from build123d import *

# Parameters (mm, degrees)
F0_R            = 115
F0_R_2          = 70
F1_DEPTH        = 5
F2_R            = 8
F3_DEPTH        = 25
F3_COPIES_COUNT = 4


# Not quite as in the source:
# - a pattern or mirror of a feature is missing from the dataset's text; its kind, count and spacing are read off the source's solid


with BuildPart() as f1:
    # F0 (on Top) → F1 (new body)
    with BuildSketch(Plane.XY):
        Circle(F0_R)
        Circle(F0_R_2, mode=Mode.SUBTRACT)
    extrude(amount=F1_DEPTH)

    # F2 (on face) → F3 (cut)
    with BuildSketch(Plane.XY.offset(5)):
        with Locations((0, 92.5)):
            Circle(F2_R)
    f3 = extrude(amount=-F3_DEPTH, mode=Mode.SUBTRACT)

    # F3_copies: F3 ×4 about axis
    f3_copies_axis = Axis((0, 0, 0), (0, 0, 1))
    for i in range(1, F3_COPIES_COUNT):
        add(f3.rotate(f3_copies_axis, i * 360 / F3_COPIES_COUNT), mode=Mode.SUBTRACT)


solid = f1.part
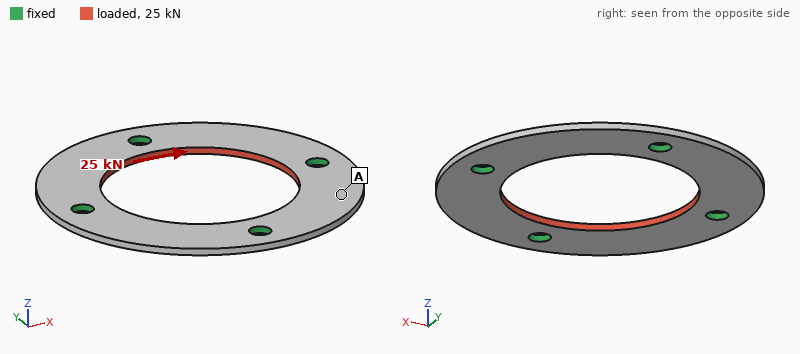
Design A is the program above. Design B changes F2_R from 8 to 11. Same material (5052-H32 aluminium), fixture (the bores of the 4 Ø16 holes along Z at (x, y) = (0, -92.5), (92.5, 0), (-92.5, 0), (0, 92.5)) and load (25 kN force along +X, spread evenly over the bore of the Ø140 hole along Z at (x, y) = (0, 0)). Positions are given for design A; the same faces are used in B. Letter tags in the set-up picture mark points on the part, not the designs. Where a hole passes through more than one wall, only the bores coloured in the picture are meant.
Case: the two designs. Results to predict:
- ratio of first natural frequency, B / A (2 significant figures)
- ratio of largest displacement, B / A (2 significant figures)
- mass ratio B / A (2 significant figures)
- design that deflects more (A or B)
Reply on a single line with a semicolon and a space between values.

1.1; 0.89; 0.97; A
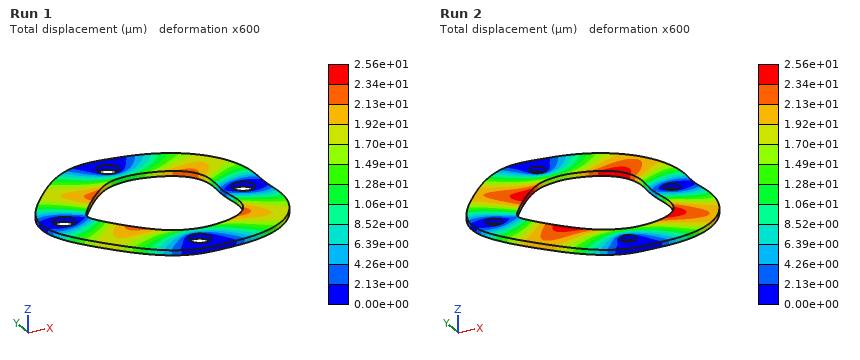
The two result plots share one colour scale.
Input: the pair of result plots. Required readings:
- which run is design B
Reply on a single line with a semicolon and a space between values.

Run 1
